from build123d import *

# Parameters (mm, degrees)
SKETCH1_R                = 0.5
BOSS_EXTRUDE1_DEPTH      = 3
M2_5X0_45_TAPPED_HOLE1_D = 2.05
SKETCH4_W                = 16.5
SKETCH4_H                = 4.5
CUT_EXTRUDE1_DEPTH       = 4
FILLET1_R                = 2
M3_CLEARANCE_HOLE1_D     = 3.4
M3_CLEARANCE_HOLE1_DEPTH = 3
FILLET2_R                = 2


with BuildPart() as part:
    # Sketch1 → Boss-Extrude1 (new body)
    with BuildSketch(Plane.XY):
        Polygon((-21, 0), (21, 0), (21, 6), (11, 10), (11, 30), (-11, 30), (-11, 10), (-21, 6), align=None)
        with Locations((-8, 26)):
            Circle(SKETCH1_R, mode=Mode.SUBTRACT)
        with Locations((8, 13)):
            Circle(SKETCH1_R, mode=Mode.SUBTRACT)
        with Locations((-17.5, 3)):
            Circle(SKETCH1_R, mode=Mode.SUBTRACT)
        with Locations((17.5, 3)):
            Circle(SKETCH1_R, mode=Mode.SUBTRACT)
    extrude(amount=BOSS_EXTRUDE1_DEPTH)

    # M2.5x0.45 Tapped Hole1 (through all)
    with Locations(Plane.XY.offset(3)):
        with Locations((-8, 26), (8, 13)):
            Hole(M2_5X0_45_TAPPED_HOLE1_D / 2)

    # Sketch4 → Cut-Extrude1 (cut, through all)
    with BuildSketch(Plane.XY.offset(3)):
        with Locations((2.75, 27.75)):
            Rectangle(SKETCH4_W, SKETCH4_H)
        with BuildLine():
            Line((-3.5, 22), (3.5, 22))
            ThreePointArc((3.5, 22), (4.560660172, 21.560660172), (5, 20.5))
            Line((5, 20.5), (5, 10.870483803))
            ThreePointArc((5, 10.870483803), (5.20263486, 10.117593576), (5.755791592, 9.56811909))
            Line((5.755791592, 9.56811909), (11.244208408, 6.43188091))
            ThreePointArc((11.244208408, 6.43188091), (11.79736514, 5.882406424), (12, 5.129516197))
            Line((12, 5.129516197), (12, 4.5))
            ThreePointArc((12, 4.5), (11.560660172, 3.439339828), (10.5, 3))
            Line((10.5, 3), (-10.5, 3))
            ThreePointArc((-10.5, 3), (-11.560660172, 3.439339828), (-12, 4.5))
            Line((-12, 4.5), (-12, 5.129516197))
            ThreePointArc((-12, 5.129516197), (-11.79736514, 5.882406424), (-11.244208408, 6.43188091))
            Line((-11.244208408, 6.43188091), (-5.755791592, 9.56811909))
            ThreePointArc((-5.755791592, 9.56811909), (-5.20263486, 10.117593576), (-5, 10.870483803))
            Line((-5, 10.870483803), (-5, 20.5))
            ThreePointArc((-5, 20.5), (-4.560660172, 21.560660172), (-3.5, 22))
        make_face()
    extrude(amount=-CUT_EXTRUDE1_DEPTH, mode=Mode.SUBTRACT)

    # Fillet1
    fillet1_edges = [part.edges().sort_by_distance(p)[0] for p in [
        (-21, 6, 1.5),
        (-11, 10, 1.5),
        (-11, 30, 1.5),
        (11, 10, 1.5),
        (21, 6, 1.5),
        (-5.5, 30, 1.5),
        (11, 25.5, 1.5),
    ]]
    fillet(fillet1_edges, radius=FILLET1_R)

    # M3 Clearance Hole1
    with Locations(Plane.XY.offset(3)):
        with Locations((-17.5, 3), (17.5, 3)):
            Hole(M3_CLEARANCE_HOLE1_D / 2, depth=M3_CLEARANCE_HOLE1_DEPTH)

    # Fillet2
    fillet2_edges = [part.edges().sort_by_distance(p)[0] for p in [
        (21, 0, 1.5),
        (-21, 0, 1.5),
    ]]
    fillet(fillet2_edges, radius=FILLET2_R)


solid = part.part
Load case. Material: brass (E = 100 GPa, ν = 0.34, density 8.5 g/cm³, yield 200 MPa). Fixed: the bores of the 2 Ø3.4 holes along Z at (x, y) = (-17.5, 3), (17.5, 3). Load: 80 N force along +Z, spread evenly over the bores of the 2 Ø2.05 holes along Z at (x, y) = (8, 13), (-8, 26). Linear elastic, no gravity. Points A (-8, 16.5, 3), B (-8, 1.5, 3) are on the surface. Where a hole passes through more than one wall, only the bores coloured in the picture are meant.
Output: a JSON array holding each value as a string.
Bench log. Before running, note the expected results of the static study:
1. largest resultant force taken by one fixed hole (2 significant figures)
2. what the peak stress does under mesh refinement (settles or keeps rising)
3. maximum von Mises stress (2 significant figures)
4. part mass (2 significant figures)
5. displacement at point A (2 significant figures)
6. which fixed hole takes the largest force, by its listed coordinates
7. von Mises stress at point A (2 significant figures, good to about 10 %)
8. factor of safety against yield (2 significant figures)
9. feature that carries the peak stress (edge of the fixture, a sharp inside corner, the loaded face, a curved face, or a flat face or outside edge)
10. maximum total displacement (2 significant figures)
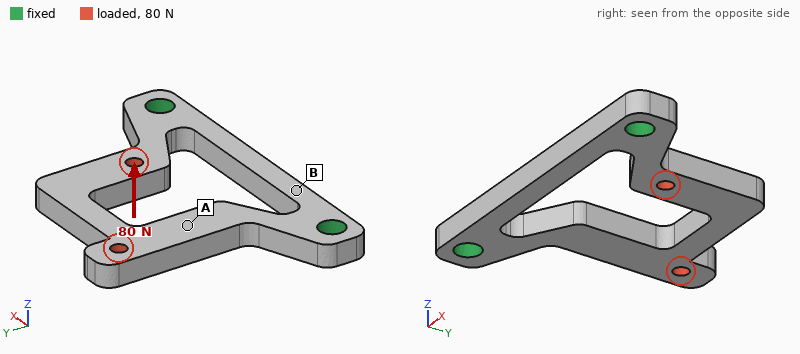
["45 N", "settles", "170 MPa", "12 g", "0.068 mm", "(17.5, 3)", "29 MPa", "1.2", "a curved face", "0.19 mm"]
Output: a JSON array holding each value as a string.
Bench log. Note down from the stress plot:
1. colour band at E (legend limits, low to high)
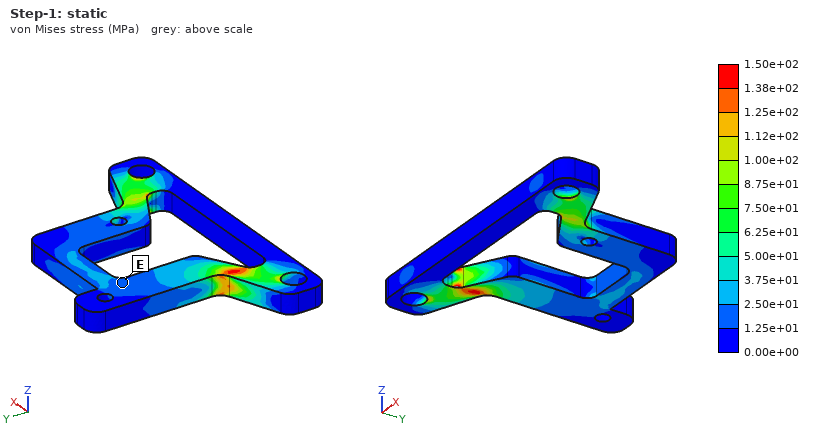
["1.25e+01 to 2.50e+01 MPa"]
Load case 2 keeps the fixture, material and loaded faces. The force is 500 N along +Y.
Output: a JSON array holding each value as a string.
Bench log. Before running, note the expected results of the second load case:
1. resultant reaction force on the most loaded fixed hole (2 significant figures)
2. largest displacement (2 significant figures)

["250 N", "12 µm"]
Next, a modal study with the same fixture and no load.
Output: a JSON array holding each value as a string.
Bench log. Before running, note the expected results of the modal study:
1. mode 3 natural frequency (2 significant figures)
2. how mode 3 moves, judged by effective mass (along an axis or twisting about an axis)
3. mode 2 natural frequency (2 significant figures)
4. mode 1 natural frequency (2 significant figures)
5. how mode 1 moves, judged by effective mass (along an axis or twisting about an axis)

["7500 Hz", "along X", "5000 Hz", "1800 Hz", "along Z"]
